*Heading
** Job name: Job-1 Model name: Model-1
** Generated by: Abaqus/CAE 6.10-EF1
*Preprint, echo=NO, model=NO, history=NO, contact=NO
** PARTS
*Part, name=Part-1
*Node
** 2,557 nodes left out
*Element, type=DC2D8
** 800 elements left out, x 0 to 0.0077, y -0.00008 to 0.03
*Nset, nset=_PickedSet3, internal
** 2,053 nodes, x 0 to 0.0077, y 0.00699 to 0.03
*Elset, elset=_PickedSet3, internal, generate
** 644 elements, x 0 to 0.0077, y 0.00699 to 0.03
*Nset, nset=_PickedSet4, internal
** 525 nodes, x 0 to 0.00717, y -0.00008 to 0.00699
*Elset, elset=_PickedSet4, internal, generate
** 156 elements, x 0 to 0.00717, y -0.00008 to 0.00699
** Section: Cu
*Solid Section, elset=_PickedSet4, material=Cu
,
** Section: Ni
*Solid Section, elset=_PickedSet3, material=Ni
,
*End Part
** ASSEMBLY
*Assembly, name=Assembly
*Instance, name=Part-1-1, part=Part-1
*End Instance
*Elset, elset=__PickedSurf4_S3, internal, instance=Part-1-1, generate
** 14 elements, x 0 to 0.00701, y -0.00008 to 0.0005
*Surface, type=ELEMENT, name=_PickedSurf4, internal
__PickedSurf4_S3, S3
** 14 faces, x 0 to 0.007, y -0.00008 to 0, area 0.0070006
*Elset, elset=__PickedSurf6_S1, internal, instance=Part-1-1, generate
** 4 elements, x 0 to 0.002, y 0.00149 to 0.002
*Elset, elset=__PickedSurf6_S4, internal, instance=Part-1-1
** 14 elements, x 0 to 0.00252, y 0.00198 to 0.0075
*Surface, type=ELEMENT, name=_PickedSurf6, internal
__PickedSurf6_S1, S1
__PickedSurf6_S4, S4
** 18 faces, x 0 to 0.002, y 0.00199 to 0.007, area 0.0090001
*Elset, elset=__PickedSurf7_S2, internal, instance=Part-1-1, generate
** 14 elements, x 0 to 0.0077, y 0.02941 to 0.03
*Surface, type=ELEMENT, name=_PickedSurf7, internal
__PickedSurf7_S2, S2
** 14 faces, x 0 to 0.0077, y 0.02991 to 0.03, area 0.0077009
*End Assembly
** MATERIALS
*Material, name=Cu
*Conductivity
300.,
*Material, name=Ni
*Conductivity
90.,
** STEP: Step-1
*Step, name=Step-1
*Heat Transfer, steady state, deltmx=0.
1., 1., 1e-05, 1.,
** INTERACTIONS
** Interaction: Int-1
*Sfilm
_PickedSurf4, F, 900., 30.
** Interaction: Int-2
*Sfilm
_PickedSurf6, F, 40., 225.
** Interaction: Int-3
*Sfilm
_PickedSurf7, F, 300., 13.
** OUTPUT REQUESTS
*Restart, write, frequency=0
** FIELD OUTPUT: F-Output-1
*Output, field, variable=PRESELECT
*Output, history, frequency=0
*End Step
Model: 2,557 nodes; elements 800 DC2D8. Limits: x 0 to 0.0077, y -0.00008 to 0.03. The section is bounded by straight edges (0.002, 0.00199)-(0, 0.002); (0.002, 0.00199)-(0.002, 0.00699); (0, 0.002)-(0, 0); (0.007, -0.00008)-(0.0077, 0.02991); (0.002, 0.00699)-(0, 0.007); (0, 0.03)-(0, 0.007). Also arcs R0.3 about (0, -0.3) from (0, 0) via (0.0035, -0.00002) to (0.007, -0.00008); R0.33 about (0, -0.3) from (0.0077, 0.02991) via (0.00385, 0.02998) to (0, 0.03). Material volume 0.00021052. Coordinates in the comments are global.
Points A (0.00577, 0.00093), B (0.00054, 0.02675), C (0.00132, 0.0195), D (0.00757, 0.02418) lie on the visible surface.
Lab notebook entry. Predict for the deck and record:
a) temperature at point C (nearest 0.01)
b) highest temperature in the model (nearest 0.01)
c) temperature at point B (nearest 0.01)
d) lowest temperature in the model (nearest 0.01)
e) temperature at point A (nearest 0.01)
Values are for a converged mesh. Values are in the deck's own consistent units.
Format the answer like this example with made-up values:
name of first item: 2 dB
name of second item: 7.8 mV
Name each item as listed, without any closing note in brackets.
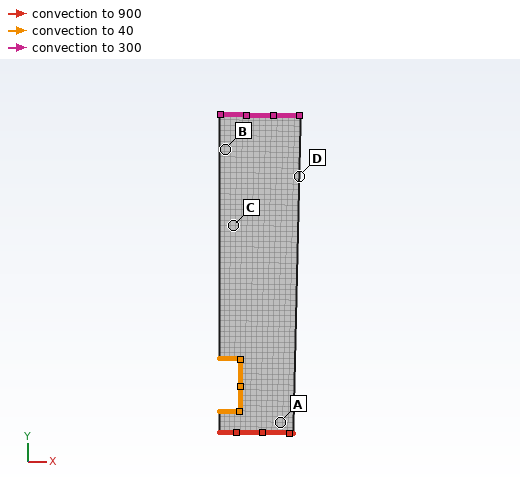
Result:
temperature at point C: 128.69
highest temperature in the model: 128.96
temperature at point B: 128.88
lowest temperature in the model: 128.01
temperature at point A: 128.81
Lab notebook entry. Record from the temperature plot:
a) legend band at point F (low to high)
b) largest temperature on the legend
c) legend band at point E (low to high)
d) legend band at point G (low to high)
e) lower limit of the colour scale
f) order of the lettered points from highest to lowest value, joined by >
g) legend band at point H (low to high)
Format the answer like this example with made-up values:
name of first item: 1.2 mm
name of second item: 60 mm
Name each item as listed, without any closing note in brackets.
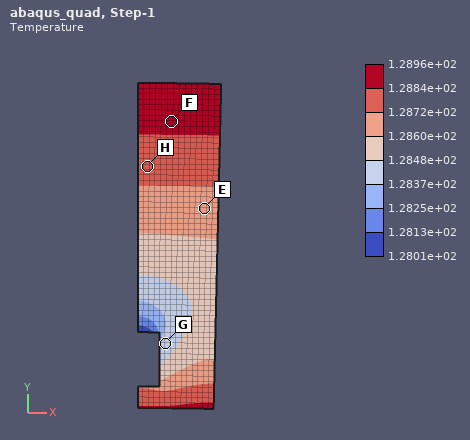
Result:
legend band at point F: 1.2884e+02 to 1.2896e+02
largest temperature on the legend: 1.2896e+02
legend band at point E: 1.2860e+02 to 1.2872e+02
legend band at point G: 1.2837e+02 to 1.2848e+02
lower limit of the colour scale: 1.2801e+02
order of the lettered points from highest to lowest value, joined by >: F > H > E > G
legend band at point H: 1.2872e+02 to 1.2884e+02
